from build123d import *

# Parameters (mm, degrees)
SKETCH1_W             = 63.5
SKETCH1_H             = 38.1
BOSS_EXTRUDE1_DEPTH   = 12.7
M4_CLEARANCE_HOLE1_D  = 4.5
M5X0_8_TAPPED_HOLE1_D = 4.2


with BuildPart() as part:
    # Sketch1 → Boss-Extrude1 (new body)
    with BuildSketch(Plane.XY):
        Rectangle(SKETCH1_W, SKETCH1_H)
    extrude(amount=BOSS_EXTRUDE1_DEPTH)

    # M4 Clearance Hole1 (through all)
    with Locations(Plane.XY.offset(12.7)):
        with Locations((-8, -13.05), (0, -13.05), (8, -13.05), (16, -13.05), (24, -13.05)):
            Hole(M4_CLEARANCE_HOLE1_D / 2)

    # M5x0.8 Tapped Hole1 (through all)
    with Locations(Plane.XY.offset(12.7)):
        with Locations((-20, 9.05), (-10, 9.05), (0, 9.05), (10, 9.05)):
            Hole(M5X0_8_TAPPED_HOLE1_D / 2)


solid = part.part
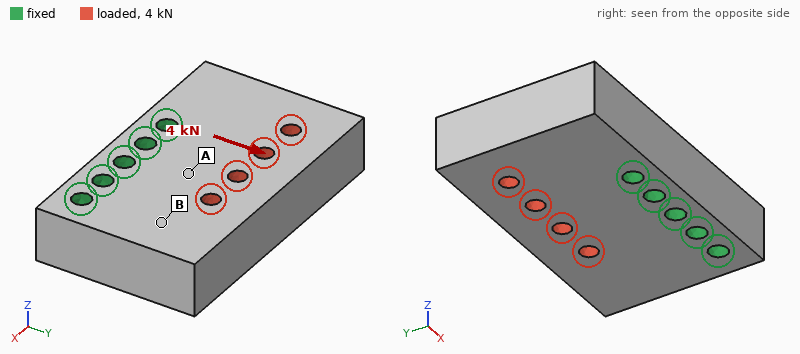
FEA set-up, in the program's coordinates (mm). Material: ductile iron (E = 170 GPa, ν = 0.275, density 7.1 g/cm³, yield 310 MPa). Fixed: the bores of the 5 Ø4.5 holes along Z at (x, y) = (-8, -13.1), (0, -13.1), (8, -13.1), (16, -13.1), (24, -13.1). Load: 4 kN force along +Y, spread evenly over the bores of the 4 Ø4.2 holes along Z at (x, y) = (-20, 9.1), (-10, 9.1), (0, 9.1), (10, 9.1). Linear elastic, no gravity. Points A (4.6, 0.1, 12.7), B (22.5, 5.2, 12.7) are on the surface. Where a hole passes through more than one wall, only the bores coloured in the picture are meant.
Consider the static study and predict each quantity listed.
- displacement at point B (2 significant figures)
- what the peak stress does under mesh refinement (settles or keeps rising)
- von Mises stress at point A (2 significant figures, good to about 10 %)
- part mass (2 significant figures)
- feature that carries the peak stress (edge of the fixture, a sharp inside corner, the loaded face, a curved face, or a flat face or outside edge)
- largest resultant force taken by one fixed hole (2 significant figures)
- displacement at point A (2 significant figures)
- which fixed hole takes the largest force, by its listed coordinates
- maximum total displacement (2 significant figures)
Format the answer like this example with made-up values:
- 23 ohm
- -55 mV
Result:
- 0.49 µm
- keeps rising
- 8.7 MPa
- 210 g
- edge of the fixture
- 2.5 kN
- 0.65 µm
- (-8, -13.1)
- 2.9 µm
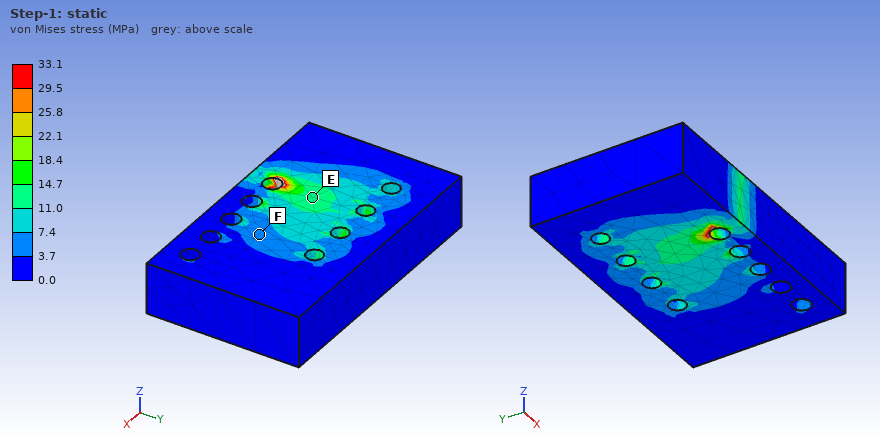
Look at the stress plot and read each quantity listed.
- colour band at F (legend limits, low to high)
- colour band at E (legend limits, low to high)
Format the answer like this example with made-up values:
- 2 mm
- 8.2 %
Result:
- 3.7 to 7.4 MPa
- 11.0 to 14.7 MPa
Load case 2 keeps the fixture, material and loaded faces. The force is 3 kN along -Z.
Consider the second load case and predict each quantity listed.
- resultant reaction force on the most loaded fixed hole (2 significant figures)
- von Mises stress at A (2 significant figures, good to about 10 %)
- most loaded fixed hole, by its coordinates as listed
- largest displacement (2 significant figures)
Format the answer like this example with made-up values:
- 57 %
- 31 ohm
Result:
- 1.4 kN
- 22 MPa
- (-8, -13.1)
- 21 µm
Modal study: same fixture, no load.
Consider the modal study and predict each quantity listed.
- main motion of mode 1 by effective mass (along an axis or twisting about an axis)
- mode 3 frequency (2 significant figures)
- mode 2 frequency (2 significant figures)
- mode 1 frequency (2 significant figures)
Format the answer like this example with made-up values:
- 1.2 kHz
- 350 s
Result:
- along Z
- 12 kHz
- 11 kHz
- 7500 Hz
